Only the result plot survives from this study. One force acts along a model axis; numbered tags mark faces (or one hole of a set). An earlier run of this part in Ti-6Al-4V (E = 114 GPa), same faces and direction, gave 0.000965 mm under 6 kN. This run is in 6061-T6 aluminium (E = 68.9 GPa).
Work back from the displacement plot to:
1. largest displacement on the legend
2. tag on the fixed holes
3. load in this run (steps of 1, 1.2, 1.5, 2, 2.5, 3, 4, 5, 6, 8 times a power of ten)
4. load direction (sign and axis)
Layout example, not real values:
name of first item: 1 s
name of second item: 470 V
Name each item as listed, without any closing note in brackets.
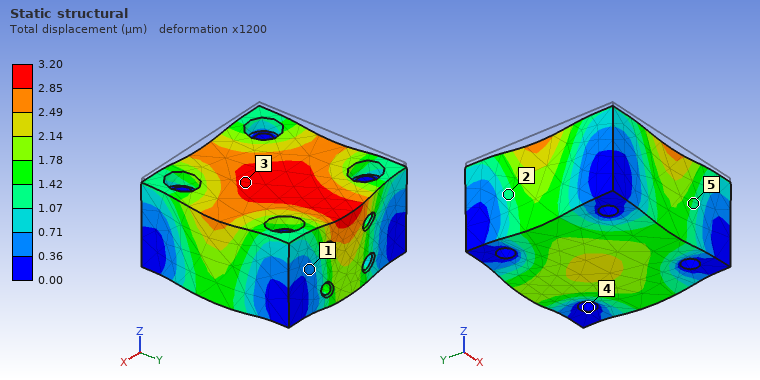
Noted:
largest displacement on the legend: 3.20 µm
tag on the fixed holes: 4
load in this run: 12 kN
load direction: -Z
